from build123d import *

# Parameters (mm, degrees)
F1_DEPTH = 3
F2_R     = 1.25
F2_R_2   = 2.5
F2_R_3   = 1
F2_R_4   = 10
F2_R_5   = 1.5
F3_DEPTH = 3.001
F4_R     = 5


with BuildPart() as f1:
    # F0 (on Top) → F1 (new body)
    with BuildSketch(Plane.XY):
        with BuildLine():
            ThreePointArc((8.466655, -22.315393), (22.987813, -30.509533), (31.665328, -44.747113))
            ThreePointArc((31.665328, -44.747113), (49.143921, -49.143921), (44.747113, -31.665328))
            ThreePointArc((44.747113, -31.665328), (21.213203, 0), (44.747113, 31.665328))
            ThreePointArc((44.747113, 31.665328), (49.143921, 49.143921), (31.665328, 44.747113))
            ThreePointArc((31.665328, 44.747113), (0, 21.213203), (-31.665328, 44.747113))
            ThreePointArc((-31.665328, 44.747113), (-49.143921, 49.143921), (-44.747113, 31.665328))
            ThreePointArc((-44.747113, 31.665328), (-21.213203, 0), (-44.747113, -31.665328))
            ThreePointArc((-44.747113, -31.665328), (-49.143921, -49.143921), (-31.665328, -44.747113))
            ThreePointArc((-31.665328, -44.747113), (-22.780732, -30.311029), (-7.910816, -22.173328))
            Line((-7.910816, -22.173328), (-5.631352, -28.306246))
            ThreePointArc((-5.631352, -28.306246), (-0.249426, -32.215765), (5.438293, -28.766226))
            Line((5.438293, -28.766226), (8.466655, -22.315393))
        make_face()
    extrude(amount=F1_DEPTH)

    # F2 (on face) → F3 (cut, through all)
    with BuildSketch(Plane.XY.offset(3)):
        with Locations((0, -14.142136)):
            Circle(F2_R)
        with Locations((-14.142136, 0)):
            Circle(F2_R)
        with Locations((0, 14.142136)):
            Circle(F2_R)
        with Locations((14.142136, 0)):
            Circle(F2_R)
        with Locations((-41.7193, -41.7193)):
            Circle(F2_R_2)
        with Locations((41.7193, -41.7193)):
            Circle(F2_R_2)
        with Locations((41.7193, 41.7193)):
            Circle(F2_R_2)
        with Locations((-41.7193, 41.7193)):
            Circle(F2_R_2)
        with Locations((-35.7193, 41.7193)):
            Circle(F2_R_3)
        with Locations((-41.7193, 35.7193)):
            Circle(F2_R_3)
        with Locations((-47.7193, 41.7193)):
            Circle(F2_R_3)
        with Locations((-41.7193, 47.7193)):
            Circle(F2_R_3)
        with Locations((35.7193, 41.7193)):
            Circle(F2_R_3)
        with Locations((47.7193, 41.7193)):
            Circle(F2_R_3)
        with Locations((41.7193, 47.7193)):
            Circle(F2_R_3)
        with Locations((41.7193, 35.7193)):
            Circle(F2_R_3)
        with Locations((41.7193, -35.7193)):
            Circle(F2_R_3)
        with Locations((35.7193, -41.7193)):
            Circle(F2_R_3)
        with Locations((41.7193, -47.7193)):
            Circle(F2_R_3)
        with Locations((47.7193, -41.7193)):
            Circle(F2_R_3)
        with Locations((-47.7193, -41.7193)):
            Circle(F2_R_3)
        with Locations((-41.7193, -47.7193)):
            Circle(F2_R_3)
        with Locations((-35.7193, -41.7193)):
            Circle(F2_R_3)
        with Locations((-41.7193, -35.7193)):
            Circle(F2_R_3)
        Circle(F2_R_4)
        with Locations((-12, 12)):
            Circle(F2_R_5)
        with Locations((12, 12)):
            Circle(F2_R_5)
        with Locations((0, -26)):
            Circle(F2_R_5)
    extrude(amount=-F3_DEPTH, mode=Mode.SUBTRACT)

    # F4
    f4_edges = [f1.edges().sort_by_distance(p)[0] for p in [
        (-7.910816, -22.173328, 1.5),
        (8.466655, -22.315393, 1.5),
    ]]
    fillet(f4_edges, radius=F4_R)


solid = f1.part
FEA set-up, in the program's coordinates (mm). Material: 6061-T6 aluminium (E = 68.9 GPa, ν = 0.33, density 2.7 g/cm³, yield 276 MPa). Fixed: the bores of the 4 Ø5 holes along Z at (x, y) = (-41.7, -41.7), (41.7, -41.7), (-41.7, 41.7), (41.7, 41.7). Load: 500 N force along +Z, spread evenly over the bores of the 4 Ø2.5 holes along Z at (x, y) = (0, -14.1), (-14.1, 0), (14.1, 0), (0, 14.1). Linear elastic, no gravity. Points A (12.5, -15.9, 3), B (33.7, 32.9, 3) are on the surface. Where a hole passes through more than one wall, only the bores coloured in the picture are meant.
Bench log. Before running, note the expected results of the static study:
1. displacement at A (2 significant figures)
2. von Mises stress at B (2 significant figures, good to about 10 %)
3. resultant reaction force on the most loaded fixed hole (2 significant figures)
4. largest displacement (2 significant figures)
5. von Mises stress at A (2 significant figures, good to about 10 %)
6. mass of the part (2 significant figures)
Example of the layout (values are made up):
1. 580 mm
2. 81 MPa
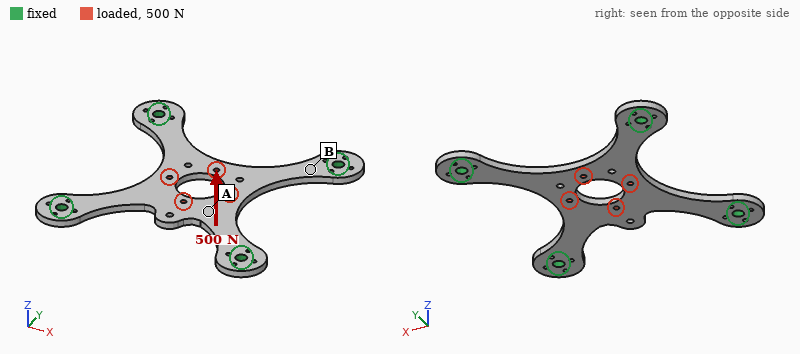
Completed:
1. 0.47 mm
2. 83 MPa
3. 130 N
4. 0.61 mm
5. 42 MPa
6. 33 g
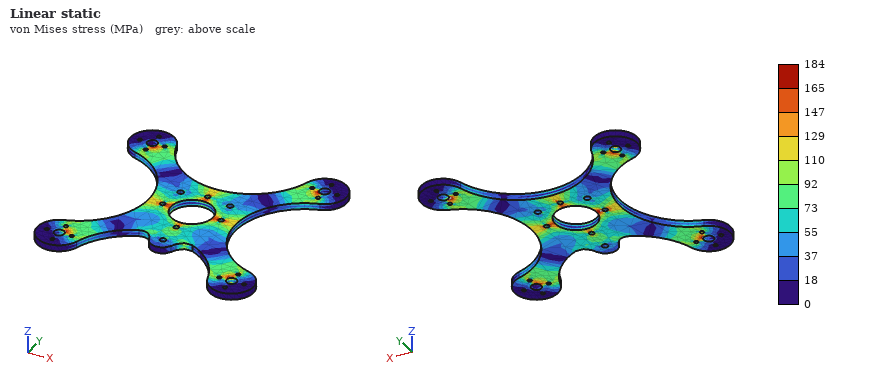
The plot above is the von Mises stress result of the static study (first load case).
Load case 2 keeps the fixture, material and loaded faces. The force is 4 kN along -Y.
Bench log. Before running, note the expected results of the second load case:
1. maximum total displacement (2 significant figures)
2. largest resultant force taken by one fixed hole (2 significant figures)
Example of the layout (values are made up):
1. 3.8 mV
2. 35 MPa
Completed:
1. 41 µm
2. 1.3 kN
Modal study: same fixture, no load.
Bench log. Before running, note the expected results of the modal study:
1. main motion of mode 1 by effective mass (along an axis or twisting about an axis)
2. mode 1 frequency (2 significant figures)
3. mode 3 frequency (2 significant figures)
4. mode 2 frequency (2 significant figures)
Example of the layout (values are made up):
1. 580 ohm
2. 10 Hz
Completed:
1. along Z
2. 1300 Hz
3. 3200 Hz
4. 2900 Hz
